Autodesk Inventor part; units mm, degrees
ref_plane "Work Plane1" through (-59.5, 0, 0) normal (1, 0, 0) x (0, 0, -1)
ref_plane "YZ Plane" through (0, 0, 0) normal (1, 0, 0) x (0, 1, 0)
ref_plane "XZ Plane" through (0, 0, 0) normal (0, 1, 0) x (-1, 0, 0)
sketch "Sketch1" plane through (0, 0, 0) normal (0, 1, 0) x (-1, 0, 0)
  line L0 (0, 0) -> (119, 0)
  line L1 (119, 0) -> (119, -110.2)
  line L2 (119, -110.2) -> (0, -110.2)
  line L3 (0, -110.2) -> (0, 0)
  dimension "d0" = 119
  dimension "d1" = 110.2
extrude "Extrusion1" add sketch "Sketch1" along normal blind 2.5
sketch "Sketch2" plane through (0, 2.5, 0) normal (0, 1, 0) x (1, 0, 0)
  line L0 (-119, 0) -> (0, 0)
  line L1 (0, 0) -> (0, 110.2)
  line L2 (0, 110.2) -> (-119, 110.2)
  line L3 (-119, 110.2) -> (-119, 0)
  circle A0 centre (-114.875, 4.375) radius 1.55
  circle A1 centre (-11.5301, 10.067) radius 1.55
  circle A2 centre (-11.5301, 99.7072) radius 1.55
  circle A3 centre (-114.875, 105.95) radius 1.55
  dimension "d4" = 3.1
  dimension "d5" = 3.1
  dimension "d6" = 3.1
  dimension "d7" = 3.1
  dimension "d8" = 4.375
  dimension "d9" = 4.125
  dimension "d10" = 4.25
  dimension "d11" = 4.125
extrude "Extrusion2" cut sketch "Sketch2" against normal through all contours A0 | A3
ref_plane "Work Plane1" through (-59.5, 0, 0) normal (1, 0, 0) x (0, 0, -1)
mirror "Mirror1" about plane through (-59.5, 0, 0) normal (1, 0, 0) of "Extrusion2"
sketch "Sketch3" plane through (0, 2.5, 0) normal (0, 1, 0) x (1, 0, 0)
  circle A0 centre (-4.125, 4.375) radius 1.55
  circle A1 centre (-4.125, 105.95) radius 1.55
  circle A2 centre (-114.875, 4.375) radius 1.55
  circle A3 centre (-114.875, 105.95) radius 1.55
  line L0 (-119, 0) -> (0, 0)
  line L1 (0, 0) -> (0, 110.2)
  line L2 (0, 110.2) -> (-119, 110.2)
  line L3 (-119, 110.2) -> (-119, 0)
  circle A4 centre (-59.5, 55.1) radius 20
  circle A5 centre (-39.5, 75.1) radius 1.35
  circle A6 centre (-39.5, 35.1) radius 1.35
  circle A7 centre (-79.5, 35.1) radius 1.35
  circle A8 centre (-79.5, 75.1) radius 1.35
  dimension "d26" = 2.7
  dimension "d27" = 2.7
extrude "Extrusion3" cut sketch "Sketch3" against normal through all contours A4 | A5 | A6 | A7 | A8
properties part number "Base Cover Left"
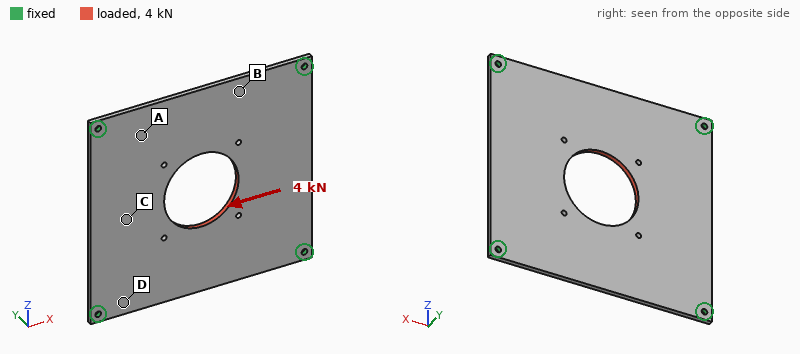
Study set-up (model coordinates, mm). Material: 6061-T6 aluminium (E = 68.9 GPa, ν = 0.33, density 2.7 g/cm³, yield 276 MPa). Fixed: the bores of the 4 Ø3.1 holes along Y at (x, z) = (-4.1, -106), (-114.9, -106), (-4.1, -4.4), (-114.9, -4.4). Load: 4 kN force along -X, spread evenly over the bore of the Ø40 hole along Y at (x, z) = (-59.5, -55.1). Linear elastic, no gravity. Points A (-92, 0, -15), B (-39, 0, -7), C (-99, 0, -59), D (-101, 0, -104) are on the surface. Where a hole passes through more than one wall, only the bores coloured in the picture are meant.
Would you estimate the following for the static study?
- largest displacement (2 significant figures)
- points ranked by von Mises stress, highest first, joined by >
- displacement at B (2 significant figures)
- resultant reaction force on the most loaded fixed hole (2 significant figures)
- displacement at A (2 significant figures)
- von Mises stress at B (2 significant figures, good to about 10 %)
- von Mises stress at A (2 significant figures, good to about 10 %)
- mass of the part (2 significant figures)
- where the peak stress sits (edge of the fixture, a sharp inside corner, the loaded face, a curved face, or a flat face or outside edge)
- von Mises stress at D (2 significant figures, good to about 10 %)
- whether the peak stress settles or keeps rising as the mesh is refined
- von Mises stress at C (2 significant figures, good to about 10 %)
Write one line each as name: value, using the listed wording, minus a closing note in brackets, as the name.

largest displacement: 22 µm
points ranked by von Mises stress, highest first, joined by >: D > A > B > C
displacement at B: 11 µm
resultant reaction force on the most loaded fixed hole: 1.1 kN
displacement at A: 11 µm
von Mises stress at B: 9.5 MPa
von Mises stress at A: 15 MPa
mass of the part: 80 g
where the peak stress sits: edge of the fixture
von Mises stress at D: 22 MPa
whether the peak stress settles or keeps rising as the mesh is refined: keeps rising
von Mises stress at C: 5.0 MPa
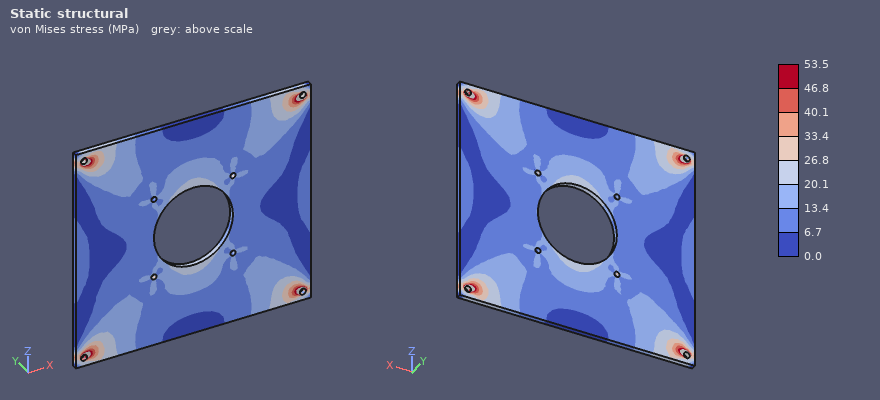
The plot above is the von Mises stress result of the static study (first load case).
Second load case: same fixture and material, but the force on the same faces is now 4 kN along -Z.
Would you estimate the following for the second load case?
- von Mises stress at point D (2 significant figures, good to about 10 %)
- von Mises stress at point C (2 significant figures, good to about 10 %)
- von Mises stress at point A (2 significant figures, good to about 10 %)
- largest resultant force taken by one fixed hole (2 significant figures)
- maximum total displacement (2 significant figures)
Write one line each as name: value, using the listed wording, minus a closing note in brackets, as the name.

von Mises stress at point D: 11 MPa
von Mises stress at point C: 14 MPa
von Mises stress at point A: 12 MPa
largest resultant force taken by one fixed hole: 1.2 kN
maximum total displacement: 25 µm
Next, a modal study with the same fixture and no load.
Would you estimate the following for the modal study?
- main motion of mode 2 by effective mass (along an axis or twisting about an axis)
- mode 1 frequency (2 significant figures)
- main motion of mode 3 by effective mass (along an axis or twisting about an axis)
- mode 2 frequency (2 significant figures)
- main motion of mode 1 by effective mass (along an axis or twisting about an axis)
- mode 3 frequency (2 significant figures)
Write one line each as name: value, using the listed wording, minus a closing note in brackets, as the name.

main motion of mode 2 by effective mass: twisting about X
mode 1 frequency: 670 Hz
main motion of mode 3 by effective mass: twisting about Z
mode 2 frequency: 1100 Hz
main motion of mode 1 by effective mass: along Y
mode 3 frequency: 1200 Hz
